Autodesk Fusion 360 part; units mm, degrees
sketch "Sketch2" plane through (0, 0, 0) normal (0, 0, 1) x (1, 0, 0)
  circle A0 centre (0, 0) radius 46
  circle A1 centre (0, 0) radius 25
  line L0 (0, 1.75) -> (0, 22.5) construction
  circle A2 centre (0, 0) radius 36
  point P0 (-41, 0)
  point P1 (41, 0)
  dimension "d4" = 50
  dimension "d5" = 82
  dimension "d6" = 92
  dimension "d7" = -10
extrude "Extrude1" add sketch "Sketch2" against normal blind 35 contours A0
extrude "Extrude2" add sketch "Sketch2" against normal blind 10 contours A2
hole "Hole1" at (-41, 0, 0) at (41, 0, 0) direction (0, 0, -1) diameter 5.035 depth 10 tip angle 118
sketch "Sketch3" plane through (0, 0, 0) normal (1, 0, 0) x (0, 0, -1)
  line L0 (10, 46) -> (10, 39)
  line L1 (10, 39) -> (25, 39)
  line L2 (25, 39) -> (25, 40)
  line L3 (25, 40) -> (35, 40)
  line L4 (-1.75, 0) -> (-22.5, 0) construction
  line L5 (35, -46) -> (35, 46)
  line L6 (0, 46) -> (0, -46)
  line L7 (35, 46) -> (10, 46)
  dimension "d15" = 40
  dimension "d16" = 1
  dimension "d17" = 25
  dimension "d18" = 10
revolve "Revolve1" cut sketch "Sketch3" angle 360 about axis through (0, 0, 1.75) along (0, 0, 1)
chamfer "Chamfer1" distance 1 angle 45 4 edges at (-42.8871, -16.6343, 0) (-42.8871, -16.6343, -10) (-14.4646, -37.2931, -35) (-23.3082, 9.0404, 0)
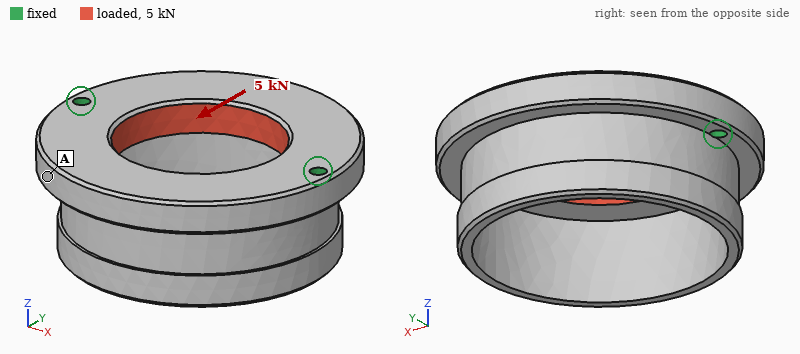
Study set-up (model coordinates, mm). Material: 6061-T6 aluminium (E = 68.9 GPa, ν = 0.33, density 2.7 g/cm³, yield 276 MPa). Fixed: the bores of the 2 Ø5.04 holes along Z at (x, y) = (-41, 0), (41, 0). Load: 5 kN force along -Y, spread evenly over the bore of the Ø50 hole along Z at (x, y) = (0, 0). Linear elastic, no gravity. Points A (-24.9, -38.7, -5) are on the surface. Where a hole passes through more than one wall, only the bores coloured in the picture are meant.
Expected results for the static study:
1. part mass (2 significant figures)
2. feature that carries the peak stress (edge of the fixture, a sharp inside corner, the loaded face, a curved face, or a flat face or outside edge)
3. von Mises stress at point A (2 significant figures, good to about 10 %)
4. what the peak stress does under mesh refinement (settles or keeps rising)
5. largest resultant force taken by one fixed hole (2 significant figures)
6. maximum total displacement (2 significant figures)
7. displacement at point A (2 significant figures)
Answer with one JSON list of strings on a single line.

["180 g", "edge of the fixture", "4.4 MPa", "keeps rising", "2.5 kN", "6.9 µm", "4.6 µm"]
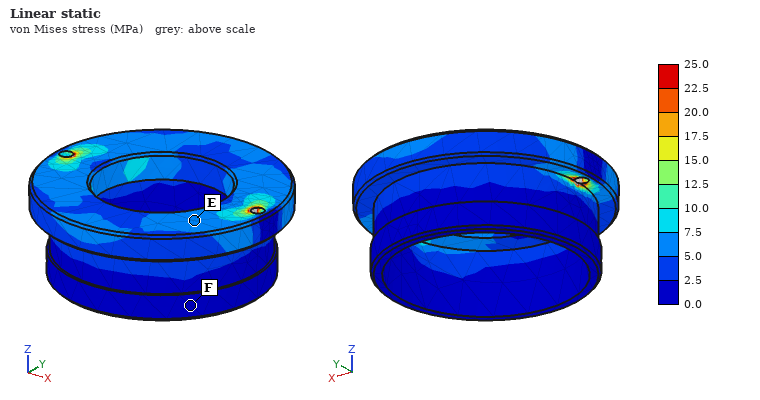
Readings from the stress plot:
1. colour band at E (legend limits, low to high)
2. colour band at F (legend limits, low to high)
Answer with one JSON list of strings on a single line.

["5.0 to 7.5 MPa", "0.0 to 2.5 MPa"]
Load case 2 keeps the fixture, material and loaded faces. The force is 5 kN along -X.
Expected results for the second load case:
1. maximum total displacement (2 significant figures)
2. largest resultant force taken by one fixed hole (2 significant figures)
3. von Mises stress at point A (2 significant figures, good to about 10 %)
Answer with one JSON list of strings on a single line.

["9.4 µm", "2.5 kN", "5.0 MPa"]
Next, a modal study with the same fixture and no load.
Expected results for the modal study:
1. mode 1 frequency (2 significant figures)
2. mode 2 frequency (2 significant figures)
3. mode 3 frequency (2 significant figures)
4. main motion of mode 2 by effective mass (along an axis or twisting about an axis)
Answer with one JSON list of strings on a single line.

["2500 Hz", "3100 Hz", "5100 Hz", "along Z"]
